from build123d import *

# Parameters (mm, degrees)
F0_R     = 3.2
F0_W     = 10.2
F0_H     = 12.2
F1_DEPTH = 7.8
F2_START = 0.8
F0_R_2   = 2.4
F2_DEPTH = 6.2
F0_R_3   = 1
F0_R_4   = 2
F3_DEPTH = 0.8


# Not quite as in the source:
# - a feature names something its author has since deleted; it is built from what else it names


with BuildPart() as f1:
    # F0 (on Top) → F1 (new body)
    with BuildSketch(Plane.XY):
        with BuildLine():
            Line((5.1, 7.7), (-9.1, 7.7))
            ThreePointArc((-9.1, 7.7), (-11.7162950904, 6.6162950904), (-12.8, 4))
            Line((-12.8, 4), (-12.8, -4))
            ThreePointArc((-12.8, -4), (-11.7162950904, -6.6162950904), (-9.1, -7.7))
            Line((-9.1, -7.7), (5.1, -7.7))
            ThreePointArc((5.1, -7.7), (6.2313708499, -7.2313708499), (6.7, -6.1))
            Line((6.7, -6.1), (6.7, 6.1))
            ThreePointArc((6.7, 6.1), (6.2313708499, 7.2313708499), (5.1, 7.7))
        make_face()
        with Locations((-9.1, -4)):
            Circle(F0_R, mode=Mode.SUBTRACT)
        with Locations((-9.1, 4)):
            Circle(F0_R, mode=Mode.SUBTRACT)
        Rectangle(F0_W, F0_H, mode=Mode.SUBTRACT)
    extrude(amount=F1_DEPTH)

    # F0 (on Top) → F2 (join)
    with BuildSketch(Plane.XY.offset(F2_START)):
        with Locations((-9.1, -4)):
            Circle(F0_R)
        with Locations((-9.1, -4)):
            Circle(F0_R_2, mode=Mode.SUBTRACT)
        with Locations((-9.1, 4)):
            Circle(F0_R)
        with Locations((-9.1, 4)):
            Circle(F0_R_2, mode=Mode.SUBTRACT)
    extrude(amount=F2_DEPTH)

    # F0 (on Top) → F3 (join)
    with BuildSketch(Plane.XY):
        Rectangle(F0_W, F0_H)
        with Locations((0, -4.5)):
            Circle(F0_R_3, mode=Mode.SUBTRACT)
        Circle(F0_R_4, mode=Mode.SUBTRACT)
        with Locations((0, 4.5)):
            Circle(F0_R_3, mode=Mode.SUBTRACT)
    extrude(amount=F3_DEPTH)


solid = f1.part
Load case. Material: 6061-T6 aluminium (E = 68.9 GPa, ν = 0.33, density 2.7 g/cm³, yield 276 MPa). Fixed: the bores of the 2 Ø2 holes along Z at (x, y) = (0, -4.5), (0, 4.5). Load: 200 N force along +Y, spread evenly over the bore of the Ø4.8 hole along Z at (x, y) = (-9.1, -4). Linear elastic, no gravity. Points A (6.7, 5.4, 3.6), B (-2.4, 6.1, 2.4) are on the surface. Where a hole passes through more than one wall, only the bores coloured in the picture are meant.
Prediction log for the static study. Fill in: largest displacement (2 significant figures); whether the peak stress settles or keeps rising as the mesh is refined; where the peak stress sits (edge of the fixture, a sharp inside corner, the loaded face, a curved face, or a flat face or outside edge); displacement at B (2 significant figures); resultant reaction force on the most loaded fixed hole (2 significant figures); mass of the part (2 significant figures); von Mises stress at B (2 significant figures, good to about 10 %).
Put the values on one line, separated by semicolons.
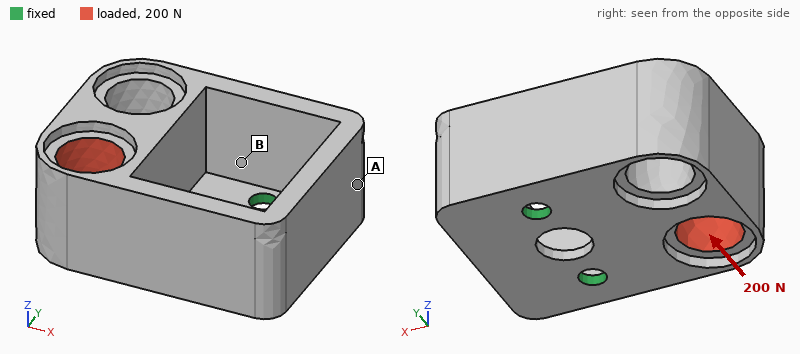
18 µm; keeps rising; edge of the fixture; 6.0 µm; 200 N; 2.9 g; 18 MPa
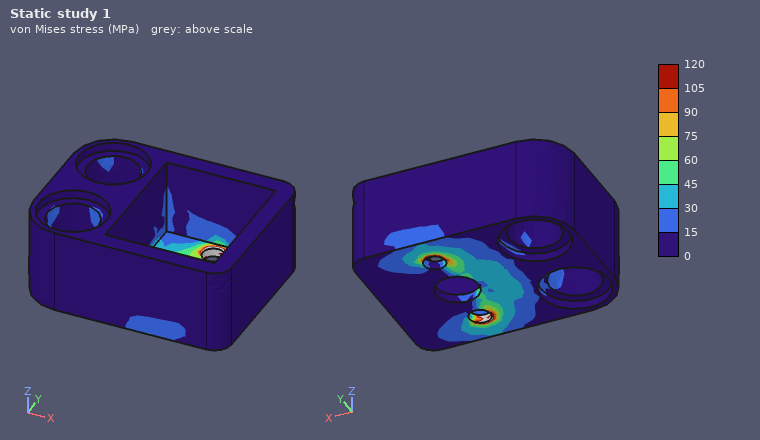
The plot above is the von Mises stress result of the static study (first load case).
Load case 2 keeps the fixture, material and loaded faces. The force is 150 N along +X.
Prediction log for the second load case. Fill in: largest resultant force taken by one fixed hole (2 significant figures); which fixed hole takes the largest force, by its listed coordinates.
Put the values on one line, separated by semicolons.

130 N; (0, -4.5)
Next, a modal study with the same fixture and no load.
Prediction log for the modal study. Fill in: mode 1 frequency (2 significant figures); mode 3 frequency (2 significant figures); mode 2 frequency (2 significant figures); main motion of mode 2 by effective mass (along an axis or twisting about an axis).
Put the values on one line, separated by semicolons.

3900 Hz; 19 kHz; 14 kHz; along Y
